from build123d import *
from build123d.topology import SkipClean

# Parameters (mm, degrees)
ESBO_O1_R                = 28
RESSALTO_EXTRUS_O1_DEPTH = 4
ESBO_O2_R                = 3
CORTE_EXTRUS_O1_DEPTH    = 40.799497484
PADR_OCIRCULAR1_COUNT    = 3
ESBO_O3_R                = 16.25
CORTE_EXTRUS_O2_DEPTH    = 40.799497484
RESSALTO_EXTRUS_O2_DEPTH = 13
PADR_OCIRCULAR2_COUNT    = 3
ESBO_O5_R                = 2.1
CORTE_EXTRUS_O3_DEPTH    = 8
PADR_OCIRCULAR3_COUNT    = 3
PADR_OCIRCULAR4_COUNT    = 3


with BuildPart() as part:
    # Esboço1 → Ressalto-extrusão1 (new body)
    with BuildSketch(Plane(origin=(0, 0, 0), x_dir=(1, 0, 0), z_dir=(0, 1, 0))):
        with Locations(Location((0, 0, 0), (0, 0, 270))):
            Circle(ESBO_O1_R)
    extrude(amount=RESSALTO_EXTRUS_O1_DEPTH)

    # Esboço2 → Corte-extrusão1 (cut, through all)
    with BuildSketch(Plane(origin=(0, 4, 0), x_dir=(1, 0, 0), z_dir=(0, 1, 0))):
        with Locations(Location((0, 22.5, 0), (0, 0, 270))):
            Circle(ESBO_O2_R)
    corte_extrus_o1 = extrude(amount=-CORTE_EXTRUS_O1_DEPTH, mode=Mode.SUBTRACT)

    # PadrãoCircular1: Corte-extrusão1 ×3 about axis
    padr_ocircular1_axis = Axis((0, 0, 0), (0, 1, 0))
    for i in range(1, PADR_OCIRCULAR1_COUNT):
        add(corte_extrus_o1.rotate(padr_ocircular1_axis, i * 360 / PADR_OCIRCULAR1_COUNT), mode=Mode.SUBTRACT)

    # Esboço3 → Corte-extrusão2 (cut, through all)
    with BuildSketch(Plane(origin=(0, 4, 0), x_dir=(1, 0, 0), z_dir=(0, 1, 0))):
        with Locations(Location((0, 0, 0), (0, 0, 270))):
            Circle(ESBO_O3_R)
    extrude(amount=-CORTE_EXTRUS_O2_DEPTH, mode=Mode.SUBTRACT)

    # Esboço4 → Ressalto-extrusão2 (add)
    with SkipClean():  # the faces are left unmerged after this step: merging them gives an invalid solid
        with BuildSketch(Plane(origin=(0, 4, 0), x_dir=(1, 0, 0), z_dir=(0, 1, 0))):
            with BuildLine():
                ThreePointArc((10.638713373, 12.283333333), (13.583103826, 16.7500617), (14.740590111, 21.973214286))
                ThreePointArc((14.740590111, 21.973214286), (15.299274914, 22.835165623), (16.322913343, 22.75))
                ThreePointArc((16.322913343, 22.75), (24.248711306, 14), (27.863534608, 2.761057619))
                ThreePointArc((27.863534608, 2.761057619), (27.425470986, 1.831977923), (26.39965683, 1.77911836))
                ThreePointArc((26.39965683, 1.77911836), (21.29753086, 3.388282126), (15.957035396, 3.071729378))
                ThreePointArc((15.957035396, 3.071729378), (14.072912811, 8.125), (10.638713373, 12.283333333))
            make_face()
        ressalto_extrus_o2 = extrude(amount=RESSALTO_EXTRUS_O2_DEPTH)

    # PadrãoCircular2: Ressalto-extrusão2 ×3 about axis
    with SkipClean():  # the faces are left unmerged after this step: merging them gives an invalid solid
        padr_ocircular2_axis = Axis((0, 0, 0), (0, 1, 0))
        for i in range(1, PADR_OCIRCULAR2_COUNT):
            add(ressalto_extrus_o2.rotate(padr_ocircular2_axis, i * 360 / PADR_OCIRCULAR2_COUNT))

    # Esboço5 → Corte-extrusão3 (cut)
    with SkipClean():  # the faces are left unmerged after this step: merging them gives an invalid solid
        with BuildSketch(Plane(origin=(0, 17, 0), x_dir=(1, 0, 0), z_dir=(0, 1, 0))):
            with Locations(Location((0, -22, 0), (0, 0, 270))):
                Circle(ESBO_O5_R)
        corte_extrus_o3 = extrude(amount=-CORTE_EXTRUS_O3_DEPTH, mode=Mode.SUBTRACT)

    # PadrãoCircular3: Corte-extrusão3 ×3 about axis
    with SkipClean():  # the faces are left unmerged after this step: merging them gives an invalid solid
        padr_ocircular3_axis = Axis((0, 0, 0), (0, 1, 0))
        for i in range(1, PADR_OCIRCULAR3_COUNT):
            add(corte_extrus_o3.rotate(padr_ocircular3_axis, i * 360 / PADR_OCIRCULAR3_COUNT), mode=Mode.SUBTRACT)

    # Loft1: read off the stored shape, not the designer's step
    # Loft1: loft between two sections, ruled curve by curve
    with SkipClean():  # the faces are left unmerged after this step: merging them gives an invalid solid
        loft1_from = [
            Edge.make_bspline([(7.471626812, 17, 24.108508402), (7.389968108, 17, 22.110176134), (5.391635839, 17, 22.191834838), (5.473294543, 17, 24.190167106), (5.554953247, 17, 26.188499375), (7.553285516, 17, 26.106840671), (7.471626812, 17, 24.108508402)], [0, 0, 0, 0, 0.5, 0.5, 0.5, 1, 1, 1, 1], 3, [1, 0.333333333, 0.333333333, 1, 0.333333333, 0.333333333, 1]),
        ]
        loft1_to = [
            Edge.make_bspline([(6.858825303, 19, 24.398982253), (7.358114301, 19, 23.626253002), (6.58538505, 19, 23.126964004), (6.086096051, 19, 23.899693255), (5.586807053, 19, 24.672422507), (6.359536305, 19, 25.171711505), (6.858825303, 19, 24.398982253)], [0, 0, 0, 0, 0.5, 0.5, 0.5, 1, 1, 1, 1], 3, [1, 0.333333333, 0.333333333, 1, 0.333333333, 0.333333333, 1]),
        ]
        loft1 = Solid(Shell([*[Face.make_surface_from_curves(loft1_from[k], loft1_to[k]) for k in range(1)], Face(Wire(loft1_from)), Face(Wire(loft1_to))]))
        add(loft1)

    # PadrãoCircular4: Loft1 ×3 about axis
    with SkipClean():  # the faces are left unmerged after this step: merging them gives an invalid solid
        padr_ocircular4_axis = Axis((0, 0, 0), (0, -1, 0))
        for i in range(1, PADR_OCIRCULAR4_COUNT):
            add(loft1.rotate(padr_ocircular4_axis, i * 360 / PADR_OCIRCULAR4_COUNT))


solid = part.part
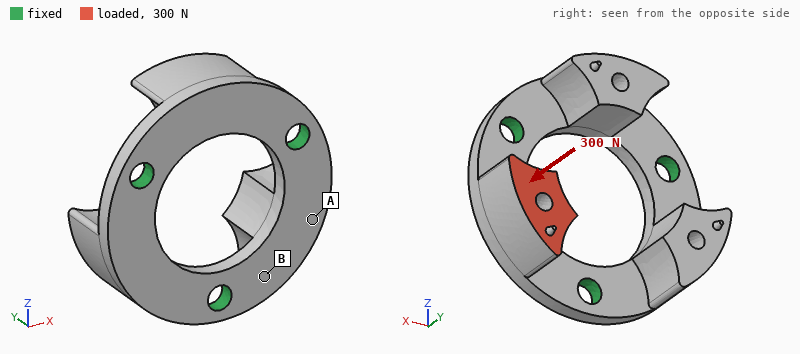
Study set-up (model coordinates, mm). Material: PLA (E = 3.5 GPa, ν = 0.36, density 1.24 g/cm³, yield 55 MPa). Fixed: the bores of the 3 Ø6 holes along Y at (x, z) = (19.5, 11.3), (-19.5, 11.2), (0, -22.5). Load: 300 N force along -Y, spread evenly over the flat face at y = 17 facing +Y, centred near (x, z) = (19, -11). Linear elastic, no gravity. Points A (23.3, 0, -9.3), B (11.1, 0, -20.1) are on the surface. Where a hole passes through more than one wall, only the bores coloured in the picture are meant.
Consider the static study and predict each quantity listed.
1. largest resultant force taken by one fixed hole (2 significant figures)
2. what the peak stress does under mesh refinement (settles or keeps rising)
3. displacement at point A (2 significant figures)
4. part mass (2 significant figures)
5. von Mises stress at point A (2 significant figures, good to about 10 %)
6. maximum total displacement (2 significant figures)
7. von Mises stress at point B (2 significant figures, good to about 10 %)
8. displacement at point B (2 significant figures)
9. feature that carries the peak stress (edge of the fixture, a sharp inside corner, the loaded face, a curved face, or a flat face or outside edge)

150 N
keeps rising
0.49 mm
17 g
6.3 MPa
0.83 mm
16 MPa
0.25 mm
edge of the fixture
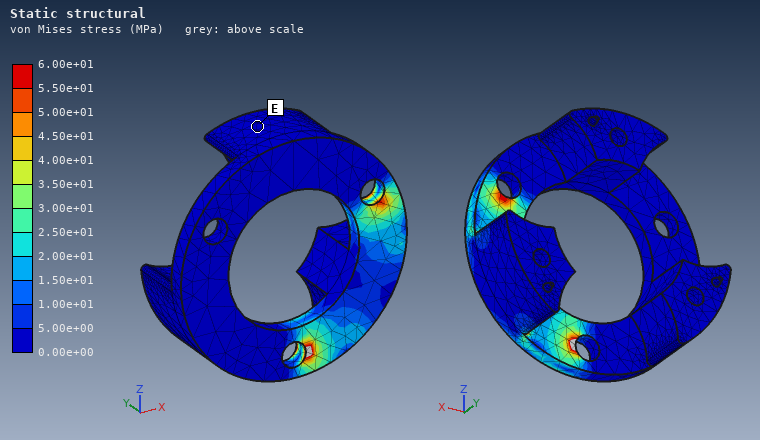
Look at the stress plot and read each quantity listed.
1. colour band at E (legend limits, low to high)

0.00e+00 to 5.00e+00 MPa
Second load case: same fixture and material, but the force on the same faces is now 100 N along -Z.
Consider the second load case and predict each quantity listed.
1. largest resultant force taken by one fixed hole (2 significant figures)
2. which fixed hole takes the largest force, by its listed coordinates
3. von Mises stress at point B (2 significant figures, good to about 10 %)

93 N
(19.5, 11.3)
9.4 MPa
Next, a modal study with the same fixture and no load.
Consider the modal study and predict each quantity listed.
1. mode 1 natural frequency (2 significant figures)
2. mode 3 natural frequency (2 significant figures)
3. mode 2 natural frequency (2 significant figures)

1500 Hz
1500 Hz
1500 Hz
